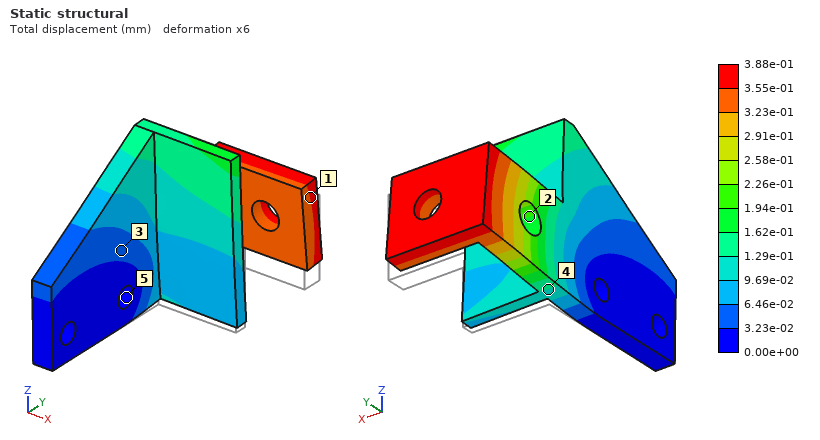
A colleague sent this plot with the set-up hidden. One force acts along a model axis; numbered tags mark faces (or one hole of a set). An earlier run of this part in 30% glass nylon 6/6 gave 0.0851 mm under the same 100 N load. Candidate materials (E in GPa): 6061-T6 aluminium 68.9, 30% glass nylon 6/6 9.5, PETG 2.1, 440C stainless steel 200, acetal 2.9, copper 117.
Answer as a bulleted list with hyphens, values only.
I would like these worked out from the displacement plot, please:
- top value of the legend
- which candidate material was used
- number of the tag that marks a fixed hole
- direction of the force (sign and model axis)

- 3.88e-01 mm
- PETG
- 5
- +Z
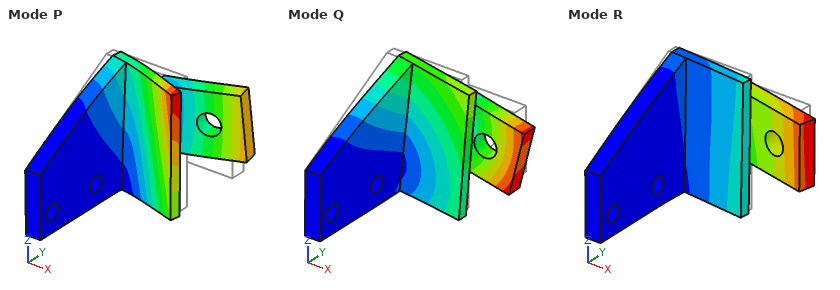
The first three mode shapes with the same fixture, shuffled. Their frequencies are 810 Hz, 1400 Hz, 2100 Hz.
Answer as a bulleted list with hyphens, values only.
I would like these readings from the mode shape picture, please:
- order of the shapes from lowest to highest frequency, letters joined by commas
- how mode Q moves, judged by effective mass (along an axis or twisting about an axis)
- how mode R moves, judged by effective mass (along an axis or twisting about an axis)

- R, Q, P
- along Z
- along X
